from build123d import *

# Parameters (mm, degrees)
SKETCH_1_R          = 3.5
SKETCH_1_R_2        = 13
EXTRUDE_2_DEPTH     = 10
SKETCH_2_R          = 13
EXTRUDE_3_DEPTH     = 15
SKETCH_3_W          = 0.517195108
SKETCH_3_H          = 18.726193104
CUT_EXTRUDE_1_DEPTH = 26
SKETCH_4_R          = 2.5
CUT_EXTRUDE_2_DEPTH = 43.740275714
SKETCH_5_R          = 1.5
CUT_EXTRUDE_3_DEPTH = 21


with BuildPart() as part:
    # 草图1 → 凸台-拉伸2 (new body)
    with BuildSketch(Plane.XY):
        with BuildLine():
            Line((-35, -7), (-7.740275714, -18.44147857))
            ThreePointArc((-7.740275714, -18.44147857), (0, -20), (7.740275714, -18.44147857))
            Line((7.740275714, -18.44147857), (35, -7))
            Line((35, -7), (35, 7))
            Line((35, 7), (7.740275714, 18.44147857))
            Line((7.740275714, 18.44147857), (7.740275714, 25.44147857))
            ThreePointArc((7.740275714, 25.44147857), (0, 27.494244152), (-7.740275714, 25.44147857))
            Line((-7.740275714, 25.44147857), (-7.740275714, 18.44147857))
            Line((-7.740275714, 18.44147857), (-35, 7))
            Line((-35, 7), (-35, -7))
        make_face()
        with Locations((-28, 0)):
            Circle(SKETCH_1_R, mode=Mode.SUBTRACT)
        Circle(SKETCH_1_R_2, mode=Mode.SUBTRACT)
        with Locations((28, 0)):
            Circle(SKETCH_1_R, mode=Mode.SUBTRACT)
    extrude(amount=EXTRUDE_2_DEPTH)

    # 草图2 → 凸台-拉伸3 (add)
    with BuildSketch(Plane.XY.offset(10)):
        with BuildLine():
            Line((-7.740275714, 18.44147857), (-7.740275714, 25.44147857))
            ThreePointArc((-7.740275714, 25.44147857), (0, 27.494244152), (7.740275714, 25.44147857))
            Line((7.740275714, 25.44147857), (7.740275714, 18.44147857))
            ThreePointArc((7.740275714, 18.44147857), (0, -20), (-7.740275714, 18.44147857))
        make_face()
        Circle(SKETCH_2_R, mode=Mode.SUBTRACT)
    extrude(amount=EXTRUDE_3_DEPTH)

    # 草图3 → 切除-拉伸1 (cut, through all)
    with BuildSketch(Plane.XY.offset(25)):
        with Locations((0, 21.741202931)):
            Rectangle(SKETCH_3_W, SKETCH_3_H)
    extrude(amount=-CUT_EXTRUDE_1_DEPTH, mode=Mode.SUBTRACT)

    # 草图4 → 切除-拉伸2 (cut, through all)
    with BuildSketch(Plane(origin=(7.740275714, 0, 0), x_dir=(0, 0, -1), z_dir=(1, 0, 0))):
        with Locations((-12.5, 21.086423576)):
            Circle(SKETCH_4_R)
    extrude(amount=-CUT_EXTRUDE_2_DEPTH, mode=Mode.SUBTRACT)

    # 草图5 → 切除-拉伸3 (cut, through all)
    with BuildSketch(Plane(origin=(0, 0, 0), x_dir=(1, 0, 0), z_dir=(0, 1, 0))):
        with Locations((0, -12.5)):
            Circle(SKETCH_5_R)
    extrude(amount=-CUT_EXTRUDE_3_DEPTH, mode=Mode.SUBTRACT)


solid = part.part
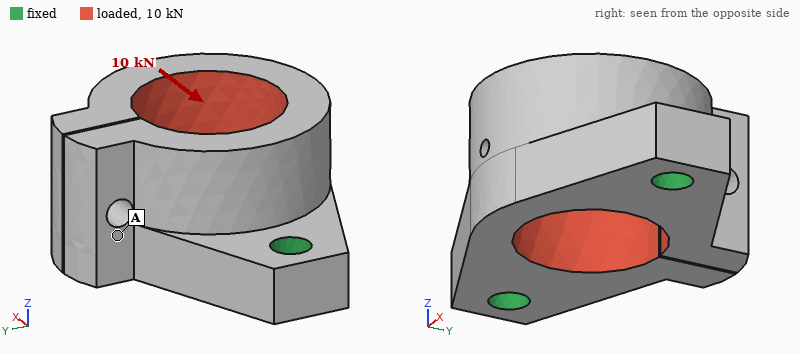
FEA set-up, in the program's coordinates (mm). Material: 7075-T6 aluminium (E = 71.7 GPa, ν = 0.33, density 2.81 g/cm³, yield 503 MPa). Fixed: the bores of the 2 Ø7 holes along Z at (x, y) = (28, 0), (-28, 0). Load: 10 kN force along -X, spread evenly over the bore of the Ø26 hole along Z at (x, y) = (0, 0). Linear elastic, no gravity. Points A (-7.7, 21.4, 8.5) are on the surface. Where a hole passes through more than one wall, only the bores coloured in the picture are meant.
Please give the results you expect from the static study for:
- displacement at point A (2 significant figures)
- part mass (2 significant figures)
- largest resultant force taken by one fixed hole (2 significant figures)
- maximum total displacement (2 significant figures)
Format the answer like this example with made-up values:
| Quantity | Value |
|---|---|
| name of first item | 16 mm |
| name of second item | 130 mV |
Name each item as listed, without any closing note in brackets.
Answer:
| Quantity | Value |
|---|---|
| displacement at point A | 46 µm |
| part mass | 76 g |
| largest resultant force taken by one fixed hole | 5.1 kN |
| maximum total displacement | 92 µm |
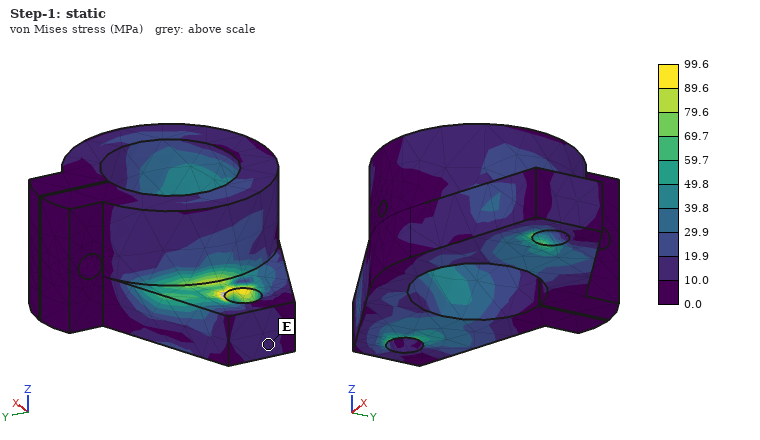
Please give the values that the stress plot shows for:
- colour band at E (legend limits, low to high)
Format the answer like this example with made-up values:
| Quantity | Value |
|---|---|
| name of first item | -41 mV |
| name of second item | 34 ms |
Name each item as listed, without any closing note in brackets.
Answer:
| Quantity | Value |
|---|---|
| colour band at E | 10.0 to 19.9 MPa |
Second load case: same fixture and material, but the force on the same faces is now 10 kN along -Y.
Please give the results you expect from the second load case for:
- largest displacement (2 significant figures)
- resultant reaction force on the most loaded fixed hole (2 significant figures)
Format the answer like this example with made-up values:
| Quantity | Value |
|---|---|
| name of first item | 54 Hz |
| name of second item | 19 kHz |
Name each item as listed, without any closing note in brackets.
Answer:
| Quantity | Value |
|---|---|
| largest displacement | 0.16 mm |
| resultant reaction force on the most loaded fixed hole | 5.9 kN |
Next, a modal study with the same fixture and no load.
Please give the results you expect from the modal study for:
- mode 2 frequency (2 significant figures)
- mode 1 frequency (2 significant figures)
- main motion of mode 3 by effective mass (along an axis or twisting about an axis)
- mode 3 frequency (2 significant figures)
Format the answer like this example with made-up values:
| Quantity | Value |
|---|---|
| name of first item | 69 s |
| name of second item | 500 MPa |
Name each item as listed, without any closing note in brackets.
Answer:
| Quantity | Value |
|---|---|
| mode 2 frequency | 5600 Hz |
| mode 1 frequency | 5600 Hz |
| main motion of mode 3 by effective mass | along Y |
| mode 3 frequency | 6200 Hz |
